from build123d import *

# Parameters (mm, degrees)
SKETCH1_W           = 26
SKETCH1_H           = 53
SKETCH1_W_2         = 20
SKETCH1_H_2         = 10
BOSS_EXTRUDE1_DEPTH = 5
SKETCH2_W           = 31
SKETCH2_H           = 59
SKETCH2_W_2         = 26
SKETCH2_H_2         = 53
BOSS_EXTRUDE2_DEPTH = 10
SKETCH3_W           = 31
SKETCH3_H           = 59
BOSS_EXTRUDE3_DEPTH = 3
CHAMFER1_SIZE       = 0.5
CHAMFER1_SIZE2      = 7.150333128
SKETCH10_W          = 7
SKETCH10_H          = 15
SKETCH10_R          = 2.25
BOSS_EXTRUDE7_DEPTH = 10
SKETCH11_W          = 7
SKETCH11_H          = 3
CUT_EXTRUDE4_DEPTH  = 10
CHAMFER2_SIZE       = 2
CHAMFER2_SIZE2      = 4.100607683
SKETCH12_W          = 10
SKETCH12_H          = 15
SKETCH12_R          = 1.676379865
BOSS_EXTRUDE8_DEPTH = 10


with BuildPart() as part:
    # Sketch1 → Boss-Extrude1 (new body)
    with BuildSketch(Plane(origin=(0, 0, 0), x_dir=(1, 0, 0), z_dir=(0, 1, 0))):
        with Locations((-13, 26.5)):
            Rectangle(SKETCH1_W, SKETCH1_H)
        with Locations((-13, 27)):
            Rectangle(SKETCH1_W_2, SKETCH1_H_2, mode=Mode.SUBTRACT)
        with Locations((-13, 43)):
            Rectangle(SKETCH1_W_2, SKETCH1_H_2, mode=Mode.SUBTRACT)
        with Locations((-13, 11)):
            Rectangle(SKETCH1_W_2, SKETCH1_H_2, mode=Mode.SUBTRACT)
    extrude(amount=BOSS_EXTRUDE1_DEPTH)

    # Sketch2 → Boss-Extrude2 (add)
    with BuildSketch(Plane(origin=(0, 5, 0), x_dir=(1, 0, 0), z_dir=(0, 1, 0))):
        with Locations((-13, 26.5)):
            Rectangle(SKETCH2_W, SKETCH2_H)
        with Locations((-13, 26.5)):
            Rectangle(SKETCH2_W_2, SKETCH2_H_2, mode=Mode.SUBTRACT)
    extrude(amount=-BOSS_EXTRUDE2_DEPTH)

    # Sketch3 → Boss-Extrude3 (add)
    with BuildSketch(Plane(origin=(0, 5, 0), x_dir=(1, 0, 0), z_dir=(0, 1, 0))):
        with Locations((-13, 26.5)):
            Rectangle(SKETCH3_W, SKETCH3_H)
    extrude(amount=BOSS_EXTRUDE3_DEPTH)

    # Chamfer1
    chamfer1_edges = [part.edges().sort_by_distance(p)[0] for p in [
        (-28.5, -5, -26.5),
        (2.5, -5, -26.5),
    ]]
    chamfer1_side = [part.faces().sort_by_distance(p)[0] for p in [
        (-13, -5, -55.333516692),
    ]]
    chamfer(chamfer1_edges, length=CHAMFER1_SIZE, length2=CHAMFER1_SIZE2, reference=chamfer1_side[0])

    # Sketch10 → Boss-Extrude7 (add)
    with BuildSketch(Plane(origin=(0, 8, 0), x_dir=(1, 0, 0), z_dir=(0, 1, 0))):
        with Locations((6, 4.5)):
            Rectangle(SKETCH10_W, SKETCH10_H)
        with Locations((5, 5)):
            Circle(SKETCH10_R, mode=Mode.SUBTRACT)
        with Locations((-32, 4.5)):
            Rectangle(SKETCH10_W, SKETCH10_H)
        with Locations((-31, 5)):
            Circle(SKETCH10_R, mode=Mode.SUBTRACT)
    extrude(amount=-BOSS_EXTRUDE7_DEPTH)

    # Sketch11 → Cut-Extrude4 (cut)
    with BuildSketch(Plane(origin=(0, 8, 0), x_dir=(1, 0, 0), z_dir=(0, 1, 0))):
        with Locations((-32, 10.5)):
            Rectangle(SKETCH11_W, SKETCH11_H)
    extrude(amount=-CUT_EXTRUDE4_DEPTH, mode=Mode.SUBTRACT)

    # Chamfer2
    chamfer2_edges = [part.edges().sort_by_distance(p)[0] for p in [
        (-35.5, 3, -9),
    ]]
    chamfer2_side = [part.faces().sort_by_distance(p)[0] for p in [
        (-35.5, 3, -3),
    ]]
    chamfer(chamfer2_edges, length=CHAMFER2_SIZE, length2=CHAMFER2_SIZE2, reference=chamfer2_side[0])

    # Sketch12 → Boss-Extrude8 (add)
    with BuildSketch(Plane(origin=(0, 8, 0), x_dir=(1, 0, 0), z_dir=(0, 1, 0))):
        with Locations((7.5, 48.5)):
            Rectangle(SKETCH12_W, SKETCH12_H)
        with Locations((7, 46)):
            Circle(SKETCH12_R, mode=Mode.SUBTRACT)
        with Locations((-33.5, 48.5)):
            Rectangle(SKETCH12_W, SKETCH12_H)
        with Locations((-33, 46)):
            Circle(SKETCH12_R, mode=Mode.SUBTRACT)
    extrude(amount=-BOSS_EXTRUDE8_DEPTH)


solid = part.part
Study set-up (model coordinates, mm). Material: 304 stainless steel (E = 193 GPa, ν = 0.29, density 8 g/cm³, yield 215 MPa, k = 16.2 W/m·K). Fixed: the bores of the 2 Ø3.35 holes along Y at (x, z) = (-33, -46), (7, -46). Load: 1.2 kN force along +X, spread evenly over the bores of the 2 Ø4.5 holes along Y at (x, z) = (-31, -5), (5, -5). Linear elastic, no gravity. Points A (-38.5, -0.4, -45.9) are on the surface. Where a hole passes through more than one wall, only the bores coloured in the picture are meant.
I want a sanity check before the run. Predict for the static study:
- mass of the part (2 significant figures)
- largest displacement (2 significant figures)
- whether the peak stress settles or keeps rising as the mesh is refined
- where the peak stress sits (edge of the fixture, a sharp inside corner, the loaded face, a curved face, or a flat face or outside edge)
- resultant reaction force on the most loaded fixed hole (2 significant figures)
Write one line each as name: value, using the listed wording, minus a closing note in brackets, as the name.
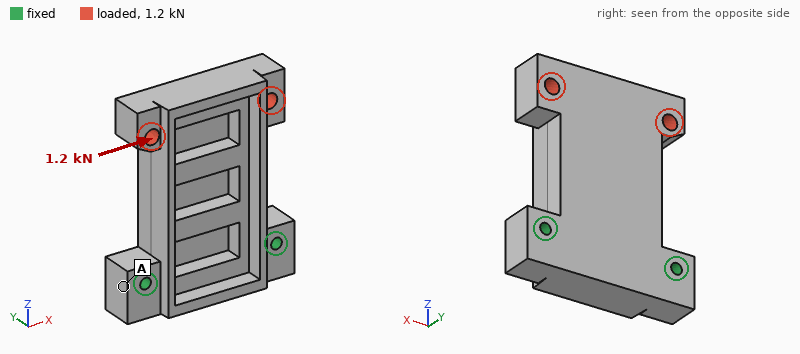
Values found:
mass of the part: 140 g
largest displacement: 37 µm
whether the peak stress settles or keeps rising as the mesh is refined: keeps rising
where the peak stress sits: edge of the fixture
resultant reaction force on the most loaded fixed hole: 1.5 kN
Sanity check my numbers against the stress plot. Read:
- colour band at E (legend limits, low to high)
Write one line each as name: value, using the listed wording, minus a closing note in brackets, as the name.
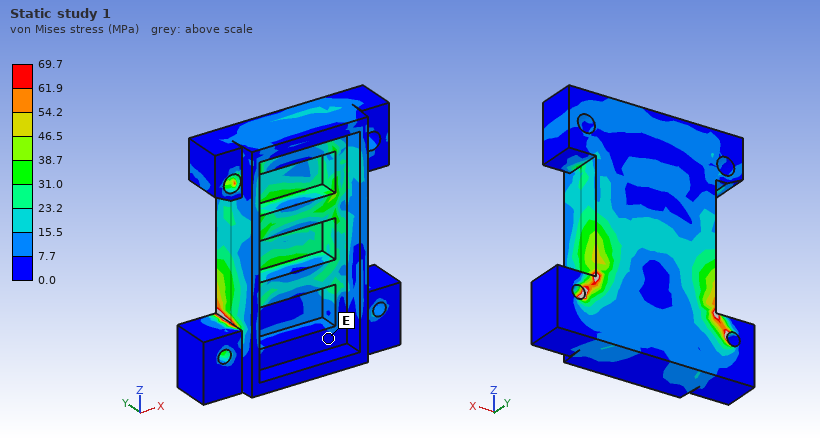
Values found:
colour band at E: 0.0 to 7.7 MPa
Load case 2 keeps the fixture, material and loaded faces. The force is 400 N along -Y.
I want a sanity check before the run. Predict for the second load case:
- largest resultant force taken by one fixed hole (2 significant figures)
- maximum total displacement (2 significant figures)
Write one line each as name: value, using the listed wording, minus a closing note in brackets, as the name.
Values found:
largest resultant force taken by one fixed hole: 200 N
maximum total displacement: 63 µm
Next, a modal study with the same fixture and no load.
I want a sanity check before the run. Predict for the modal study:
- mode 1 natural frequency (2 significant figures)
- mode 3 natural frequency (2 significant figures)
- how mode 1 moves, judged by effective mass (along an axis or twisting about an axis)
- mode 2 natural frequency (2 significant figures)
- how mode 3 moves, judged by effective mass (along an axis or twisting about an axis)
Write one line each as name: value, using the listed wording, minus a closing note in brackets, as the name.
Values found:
mode 1 natural frequency: 1900 Hz
mode 3 natural frequency: 6000 Hz
how mode 1 moves, judged by effective mass: along Y
mode 2 natural frequency: 3600 Hz
how mode 3 moves, judged by effective mass: along X
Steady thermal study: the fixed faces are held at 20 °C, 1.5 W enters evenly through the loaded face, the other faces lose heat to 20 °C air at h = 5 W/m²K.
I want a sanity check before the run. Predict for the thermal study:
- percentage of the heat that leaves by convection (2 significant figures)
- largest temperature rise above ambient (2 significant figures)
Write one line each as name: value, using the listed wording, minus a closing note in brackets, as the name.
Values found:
percentage of the heat that leaves by convection: 30 %
largest temperature rise above ambient: 23 K
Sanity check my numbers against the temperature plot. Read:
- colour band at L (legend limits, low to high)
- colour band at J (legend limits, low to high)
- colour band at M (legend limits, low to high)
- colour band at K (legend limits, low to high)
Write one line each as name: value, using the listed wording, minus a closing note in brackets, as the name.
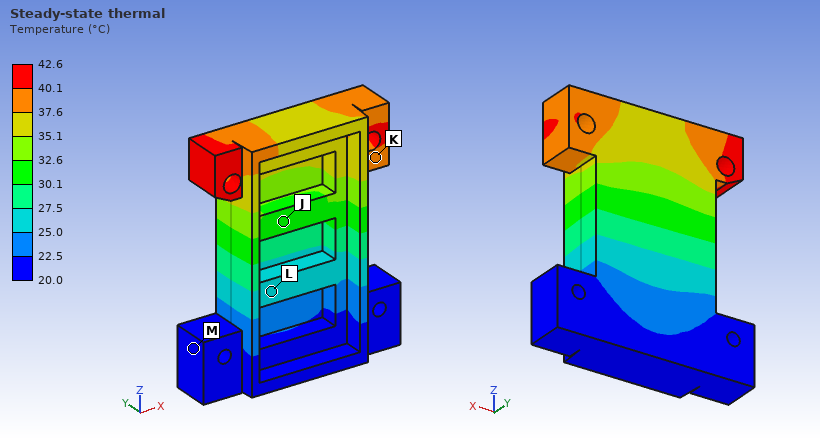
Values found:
colour band at L: 25.0 to 27.5 °C
colour band at J: 30.1 to 32.6 °C
colour band at M: 20.0 to 22.5 °C
colour band at K: 37.6 to 40.1 °C
